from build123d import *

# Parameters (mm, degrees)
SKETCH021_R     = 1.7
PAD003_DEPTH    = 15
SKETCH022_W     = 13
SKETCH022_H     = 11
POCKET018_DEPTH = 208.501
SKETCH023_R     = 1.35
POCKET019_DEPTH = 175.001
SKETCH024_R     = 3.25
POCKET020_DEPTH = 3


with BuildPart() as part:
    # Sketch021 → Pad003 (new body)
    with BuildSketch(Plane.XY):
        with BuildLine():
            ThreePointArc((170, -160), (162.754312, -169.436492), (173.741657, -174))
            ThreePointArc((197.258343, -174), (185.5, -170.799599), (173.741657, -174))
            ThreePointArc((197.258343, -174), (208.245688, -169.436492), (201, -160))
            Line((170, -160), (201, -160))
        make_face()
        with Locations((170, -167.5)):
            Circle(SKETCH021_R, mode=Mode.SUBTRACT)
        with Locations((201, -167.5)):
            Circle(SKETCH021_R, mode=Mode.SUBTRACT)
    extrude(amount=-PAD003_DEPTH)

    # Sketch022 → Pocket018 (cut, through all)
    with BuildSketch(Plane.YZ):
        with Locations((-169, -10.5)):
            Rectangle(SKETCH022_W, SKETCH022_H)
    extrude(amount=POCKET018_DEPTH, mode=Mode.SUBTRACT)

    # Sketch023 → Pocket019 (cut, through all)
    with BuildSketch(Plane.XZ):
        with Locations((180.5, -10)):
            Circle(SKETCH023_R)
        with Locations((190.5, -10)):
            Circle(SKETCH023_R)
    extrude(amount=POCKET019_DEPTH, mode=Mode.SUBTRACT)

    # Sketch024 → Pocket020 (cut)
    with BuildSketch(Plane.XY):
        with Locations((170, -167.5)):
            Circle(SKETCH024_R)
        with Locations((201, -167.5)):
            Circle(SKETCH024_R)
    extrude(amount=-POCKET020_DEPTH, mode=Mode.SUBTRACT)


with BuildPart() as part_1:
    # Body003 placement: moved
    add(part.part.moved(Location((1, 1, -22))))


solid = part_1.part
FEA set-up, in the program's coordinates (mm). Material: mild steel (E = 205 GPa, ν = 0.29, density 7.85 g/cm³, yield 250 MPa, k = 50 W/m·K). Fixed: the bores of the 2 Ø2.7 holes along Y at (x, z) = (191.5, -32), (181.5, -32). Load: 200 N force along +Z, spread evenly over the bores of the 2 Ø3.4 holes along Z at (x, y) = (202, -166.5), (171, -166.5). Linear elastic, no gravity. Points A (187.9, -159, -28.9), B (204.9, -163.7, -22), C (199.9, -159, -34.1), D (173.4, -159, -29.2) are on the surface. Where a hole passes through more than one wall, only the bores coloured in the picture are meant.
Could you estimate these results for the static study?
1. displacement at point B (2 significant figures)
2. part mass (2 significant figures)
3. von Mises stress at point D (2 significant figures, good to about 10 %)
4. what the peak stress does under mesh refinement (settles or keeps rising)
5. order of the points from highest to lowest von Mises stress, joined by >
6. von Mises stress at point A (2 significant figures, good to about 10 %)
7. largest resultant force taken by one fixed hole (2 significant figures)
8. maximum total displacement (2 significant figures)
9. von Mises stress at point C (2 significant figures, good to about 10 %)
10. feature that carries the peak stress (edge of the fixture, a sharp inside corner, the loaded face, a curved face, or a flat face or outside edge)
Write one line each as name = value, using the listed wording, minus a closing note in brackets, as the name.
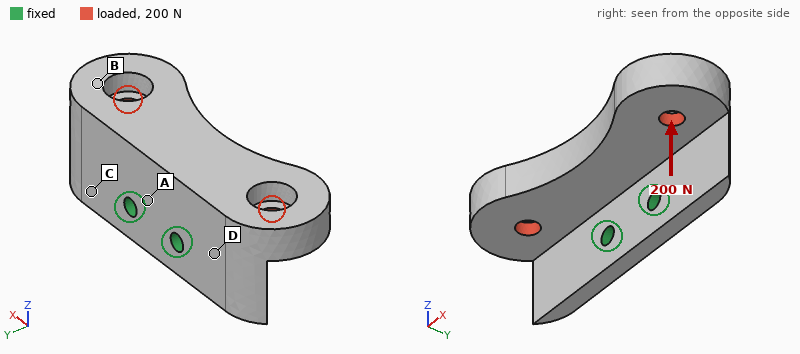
displacement at point B = 8.3 µm
part mass = 28 g
von Mises stress at point D = 19 MPa
what the peak stress does under mesh refinement = keeps rising
order of the points from highest to lowest von Mises stress, joined by > = A > D > C > B
von Mises stress at point A = 33 MPa
largest resultant force taken by one fixed hole = 110 N
maximum total displacement = 16 µm
von Mises stress at point C = 11 MPa
feature that carries the peak stress = edge of the fixture
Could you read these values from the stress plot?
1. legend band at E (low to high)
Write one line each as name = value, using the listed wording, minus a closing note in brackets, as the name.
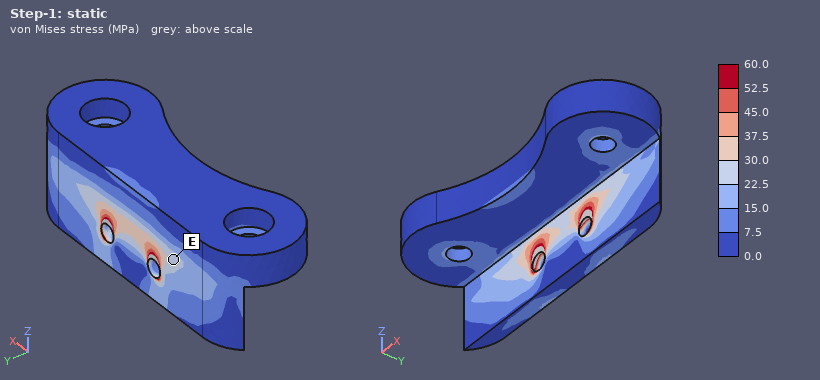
legend band at E = 22.5 to 30.0 MPa
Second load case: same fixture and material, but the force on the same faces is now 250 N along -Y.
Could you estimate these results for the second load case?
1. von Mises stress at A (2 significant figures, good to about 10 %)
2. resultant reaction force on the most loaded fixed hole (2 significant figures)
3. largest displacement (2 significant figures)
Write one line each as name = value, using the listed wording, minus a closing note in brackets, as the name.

von Mises stress at A = 22 MPa
resultant reaction force on the most loaded fixed hole = 130 N
largest displacement = 10 µm
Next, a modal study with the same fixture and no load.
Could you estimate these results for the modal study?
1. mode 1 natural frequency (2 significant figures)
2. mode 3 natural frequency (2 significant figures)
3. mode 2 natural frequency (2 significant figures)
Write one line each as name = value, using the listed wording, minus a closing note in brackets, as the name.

mode 1 natural frequency = 4800 Hz
mode 3 natural frequency = 10 kHz
mode 2 natural frequency = 5900 Hz
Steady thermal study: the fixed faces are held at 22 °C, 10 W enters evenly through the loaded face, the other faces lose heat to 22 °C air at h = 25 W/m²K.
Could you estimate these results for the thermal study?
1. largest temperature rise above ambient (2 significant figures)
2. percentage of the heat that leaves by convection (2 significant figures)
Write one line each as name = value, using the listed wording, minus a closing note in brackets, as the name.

largest temperature rise above ambient = 37 K
percentage of the heat that leaves by convection = 13 %
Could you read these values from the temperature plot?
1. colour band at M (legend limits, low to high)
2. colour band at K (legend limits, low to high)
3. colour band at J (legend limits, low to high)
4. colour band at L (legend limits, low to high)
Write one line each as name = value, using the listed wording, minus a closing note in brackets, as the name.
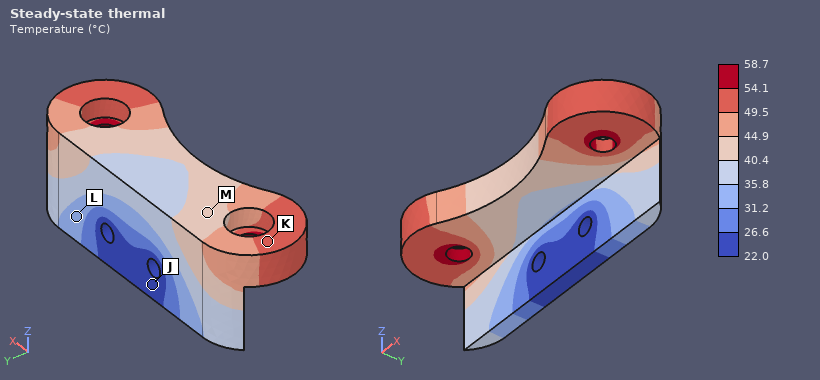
colour band at M = 40.4 to 44.9 °C
colour band at K = 49.5 to 54.1 °C
colour band at J = 22.0 to 26.6 °C
colour band at L = 31.2 to 35.8 °C
